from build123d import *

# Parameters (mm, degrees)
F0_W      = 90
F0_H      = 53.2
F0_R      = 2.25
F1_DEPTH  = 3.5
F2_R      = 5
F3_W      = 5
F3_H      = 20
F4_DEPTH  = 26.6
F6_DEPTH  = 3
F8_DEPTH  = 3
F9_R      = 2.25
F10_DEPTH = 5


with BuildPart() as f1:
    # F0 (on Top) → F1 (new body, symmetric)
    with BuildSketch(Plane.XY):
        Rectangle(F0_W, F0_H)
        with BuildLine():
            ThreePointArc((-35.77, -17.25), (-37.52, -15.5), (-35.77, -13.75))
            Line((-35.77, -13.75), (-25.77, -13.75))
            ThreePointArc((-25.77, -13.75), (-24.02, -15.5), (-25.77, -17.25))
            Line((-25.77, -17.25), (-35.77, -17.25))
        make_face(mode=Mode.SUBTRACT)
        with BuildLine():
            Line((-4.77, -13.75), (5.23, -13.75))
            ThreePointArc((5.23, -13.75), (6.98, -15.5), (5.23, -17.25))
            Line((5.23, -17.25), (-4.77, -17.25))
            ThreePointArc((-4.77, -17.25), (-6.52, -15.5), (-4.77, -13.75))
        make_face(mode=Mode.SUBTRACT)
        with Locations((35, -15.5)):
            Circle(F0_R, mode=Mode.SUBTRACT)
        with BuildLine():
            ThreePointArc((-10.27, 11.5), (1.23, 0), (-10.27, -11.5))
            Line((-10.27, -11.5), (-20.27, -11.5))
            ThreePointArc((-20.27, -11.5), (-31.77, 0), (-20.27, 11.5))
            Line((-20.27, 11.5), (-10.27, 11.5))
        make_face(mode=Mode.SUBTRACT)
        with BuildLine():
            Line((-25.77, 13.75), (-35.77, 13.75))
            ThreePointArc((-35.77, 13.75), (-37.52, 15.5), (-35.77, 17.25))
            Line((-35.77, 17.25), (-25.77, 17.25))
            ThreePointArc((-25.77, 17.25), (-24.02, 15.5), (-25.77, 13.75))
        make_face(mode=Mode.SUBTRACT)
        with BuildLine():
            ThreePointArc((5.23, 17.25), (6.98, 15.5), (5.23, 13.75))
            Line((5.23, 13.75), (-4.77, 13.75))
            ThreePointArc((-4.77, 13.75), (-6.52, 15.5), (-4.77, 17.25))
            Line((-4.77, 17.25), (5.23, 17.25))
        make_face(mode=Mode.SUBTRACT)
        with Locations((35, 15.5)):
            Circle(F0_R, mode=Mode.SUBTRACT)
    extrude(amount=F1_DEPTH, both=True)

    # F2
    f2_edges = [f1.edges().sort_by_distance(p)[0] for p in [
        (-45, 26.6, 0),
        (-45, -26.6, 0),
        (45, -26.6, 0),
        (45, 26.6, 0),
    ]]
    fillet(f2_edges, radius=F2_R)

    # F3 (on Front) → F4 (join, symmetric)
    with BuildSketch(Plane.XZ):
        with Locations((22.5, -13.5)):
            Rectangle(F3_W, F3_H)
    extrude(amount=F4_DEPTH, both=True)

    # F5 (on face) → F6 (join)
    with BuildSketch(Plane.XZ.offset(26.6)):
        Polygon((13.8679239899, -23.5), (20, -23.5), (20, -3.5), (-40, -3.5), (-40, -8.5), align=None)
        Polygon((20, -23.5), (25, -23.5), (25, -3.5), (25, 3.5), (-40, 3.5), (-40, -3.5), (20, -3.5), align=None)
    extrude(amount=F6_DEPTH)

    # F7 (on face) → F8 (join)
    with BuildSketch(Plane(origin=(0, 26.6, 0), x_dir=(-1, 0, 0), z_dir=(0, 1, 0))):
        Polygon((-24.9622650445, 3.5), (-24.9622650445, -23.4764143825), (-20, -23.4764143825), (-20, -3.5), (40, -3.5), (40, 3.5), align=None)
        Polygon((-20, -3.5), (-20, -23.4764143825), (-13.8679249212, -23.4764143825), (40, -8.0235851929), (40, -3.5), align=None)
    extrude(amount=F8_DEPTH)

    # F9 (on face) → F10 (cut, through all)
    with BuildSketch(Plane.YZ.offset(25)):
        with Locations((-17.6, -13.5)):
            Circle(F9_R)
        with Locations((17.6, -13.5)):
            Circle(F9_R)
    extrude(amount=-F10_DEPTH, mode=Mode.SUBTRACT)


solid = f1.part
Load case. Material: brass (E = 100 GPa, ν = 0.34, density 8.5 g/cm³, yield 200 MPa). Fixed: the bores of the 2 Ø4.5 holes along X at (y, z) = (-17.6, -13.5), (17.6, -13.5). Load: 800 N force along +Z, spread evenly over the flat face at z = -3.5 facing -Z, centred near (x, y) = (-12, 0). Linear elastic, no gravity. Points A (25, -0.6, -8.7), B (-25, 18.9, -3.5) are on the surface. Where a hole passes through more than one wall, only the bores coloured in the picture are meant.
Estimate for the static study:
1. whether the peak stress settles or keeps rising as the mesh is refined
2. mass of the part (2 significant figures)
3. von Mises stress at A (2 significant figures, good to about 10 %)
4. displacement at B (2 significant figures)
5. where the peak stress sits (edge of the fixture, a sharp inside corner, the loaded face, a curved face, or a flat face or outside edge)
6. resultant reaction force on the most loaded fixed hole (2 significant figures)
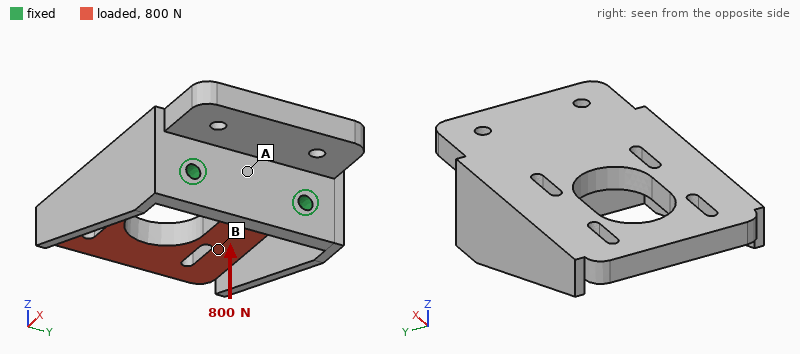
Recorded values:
keeps rising
350 g
32 MPa
0.15 mm
edge of the fixture
400 N
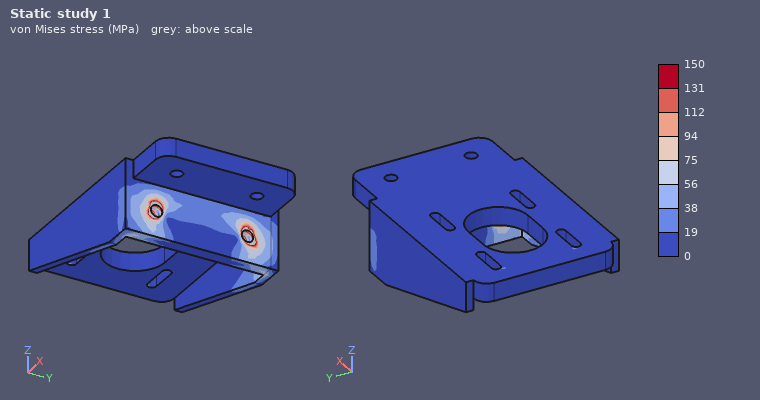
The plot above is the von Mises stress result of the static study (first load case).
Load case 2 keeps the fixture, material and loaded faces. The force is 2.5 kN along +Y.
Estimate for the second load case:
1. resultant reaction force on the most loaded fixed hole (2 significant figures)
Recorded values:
2.5 kN
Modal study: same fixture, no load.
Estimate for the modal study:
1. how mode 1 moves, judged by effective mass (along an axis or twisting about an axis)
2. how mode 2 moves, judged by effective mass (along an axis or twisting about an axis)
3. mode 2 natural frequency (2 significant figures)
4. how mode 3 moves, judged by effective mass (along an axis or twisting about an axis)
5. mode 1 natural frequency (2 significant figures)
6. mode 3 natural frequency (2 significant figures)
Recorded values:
along Z
along Y
1500 Hz
along Y
800 Hz
2800 Hz
